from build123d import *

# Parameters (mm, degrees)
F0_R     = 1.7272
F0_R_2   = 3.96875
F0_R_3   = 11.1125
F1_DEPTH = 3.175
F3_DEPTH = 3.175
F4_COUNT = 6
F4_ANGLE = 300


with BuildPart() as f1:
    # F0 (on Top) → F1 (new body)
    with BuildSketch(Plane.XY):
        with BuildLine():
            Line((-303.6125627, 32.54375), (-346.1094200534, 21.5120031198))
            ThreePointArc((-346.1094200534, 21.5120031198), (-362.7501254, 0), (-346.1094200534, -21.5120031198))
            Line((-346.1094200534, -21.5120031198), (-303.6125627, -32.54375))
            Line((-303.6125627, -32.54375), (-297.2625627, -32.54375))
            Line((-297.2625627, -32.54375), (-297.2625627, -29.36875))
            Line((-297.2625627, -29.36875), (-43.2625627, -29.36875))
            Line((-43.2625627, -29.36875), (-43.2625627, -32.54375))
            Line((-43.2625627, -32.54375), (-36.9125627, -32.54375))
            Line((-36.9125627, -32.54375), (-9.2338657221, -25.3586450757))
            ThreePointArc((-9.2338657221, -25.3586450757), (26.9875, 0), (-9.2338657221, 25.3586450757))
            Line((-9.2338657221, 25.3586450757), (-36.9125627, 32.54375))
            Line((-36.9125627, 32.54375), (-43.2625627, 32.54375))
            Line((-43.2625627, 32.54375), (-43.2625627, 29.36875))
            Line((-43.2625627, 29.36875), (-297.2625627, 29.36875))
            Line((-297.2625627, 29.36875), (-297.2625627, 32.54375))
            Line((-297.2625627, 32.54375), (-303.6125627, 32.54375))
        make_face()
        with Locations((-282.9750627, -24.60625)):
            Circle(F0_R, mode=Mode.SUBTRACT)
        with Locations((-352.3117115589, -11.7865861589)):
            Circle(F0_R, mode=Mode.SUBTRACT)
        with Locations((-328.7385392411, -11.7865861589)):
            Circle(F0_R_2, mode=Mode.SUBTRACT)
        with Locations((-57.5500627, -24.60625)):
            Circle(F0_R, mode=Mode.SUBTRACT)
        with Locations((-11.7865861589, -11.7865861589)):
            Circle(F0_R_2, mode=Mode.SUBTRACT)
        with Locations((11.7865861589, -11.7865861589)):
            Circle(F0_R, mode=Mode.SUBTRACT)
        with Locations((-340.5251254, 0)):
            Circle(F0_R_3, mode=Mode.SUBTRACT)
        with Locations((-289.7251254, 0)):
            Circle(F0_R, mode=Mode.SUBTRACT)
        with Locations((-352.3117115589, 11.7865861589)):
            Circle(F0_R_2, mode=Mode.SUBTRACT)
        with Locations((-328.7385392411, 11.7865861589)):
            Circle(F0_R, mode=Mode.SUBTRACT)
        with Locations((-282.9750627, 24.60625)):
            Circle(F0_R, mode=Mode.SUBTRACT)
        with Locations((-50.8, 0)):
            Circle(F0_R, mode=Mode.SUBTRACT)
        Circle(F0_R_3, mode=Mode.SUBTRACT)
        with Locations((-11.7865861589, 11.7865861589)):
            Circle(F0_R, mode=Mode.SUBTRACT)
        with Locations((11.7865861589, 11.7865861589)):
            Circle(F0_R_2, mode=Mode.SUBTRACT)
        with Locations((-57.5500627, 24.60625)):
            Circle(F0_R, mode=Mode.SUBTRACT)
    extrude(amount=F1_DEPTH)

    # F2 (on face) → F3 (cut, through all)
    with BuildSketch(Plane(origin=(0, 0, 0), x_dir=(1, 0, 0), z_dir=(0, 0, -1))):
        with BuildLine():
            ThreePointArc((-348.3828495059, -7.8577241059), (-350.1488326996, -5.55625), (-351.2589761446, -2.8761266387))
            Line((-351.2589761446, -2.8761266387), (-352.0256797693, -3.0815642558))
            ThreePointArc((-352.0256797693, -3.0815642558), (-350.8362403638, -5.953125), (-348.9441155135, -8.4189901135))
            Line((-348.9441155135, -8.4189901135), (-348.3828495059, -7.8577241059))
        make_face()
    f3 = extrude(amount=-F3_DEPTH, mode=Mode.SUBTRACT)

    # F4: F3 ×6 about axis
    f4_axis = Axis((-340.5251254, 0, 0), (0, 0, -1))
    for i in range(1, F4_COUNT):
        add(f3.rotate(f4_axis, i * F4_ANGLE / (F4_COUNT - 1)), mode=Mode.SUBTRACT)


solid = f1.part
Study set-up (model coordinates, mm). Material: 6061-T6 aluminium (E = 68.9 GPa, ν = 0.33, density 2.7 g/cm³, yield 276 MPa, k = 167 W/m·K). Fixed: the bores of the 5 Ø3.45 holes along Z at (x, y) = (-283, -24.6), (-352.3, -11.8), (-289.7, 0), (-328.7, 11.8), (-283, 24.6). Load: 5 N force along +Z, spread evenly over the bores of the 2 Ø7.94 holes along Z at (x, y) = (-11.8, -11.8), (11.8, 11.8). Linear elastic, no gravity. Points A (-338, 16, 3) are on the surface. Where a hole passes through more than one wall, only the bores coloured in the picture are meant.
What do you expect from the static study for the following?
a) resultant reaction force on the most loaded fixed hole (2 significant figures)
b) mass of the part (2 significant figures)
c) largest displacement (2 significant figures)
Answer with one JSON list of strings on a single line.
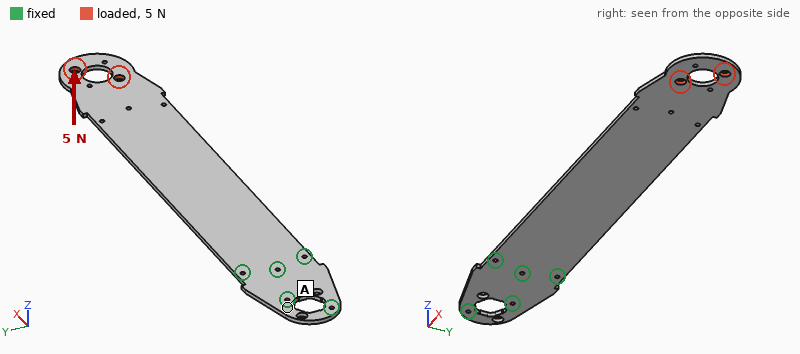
["9.3 N", "180 g", "4.1 mm"]
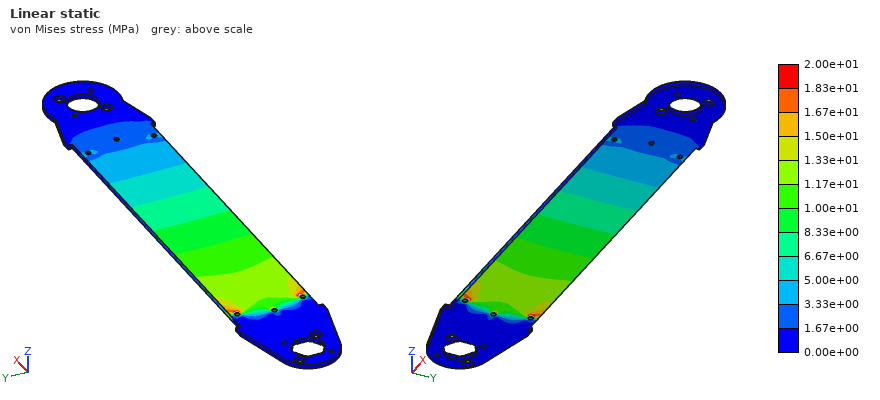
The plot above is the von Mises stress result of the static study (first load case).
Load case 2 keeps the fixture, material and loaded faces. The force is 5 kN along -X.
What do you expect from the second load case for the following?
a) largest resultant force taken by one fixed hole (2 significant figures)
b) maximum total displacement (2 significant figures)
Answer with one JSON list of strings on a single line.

["1.6 kN", "0.14 mm"]
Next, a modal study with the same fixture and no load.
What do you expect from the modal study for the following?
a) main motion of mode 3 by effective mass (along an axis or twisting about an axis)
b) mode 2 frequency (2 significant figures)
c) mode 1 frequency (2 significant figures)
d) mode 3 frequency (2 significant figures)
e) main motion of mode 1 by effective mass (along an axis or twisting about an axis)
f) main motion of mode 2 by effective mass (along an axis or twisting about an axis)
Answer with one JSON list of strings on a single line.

["twisting about X", "180 Hz", "30 Hz", "300 Hz", "along Z", "along Z"]
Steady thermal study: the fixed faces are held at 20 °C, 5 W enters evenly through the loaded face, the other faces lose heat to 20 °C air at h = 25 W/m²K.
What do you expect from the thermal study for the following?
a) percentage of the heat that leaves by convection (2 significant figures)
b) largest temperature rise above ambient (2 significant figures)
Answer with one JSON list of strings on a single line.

["90 %", "17 K"]
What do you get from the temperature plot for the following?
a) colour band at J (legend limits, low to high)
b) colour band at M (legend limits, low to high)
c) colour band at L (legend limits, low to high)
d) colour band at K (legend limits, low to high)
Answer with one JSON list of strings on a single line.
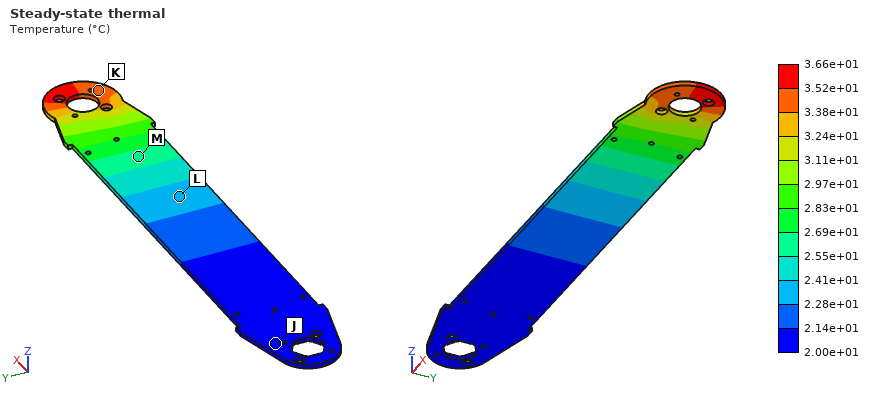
["2.00e+01 to 2.14e+01 °C", "2.55e+01 to 2.69e+01 °C", "2.28e+01 to 2.41e+01 °C", "3.38e+01 to 3.52e+01 °C"]
